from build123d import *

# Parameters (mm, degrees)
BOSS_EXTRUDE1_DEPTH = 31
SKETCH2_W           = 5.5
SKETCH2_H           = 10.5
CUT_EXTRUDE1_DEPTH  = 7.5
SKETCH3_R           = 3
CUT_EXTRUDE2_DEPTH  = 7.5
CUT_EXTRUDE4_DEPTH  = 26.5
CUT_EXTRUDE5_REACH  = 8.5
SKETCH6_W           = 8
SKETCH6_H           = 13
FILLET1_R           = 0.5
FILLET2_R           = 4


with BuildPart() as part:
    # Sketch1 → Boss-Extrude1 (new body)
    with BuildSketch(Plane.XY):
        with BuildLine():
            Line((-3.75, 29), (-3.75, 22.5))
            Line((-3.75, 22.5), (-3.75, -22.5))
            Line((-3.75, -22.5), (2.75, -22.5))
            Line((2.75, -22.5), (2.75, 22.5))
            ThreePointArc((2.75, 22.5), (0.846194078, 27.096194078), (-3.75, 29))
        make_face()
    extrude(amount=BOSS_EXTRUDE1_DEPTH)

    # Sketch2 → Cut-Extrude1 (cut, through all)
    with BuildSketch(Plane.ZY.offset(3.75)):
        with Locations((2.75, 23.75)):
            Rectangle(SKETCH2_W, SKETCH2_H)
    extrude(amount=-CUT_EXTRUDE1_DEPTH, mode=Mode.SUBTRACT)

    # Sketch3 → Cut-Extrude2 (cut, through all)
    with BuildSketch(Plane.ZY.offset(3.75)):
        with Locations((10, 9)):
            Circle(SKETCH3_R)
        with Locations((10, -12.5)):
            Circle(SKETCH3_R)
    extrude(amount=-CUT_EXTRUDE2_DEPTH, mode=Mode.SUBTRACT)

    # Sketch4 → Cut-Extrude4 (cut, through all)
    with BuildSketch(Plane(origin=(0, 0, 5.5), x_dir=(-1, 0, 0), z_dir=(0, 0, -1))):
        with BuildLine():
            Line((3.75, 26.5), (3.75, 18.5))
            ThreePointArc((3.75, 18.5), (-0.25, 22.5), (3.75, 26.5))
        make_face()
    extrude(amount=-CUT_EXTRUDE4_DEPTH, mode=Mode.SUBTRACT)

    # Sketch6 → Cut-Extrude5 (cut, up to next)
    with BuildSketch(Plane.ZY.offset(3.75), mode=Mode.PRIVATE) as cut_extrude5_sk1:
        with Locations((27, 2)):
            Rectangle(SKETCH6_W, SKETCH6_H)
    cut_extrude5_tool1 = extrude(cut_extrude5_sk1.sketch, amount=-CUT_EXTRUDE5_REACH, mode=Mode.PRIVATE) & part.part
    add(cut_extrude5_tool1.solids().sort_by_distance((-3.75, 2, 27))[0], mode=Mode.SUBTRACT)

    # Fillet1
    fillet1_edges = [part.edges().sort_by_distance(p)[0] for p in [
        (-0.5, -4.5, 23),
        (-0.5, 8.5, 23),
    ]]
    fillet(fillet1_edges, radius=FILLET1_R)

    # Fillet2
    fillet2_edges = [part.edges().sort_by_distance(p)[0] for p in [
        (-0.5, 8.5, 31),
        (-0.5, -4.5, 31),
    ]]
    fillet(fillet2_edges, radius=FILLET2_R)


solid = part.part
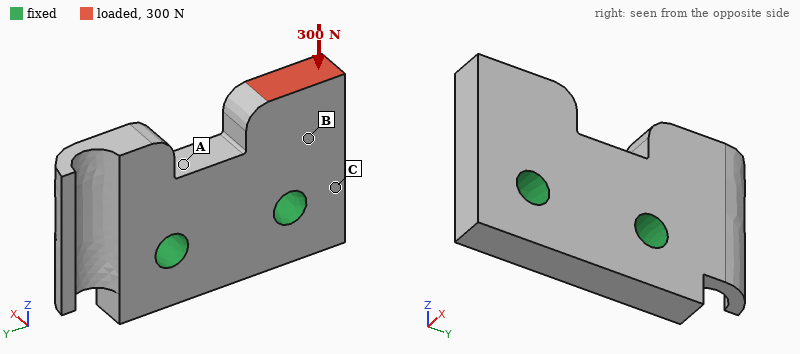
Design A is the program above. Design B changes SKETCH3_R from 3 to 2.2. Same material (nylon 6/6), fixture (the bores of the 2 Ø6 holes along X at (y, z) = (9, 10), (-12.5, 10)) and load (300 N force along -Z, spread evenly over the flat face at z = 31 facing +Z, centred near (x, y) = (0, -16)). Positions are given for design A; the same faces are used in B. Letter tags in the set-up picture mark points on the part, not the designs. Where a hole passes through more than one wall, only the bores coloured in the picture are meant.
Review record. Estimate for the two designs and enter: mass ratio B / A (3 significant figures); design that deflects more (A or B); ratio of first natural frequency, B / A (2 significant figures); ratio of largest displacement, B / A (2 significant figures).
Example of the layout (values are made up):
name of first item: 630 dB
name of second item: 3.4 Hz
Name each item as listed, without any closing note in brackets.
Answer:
mass ratio B / A: 1.02
design that deflects more: B
ratio of first natural frequency, B / A: 0.93
ratio of largest displacement, B / A: 1.1
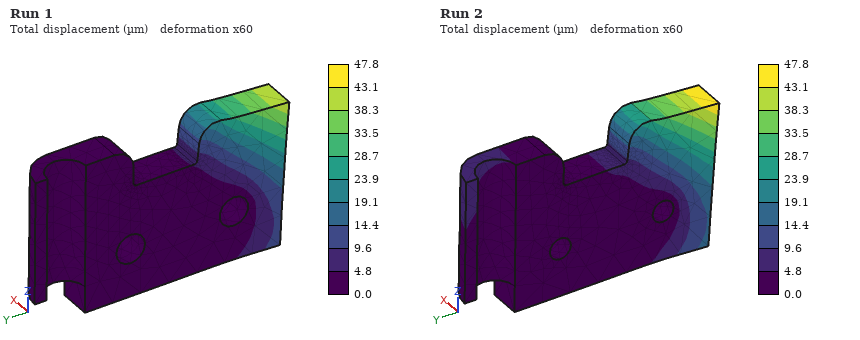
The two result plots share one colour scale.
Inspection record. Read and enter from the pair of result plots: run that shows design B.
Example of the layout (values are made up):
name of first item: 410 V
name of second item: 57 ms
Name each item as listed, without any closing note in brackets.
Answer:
run that shows design B: Run 2
